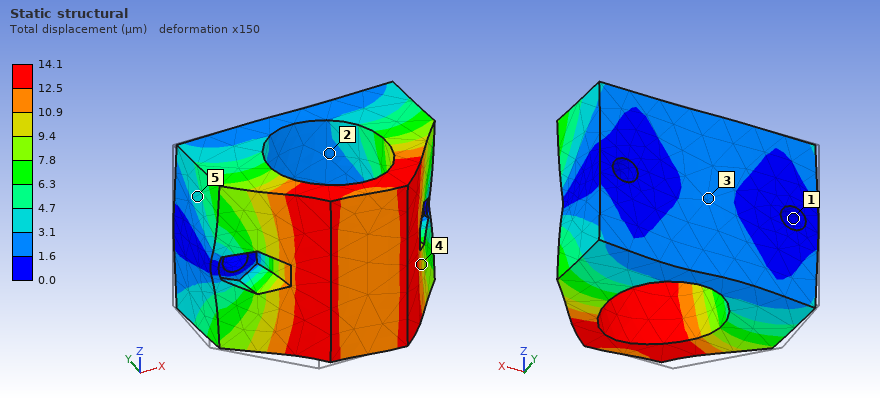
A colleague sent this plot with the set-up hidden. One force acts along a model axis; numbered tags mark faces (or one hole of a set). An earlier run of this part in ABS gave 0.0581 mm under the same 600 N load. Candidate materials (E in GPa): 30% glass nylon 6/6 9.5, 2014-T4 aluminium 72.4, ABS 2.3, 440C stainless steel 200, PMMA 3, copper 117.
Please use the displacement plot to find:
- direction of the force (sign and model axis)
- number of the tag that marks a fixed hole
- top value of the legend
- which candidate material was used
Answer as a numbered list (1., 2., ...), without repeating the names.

1. +X
2. 1
3. 14.1 µm
4. 30% glass nylon 6/6
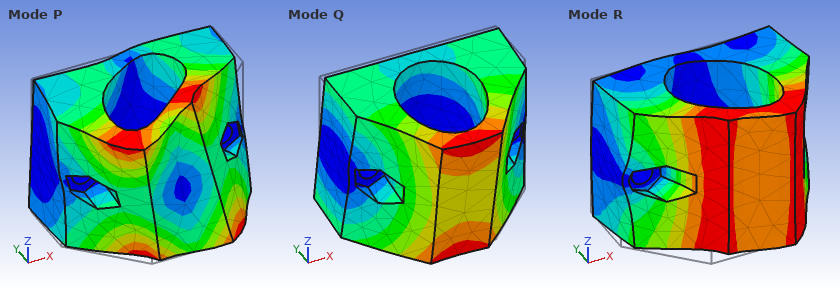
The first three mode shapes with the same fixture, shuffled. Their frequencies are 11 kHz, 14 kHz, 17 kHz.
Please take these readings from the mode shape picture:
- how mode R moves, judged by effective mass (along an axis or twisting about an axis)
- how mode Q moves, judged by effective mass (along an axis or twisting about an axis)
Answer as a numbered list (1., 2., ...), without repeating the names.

1. along X
2. along Z
